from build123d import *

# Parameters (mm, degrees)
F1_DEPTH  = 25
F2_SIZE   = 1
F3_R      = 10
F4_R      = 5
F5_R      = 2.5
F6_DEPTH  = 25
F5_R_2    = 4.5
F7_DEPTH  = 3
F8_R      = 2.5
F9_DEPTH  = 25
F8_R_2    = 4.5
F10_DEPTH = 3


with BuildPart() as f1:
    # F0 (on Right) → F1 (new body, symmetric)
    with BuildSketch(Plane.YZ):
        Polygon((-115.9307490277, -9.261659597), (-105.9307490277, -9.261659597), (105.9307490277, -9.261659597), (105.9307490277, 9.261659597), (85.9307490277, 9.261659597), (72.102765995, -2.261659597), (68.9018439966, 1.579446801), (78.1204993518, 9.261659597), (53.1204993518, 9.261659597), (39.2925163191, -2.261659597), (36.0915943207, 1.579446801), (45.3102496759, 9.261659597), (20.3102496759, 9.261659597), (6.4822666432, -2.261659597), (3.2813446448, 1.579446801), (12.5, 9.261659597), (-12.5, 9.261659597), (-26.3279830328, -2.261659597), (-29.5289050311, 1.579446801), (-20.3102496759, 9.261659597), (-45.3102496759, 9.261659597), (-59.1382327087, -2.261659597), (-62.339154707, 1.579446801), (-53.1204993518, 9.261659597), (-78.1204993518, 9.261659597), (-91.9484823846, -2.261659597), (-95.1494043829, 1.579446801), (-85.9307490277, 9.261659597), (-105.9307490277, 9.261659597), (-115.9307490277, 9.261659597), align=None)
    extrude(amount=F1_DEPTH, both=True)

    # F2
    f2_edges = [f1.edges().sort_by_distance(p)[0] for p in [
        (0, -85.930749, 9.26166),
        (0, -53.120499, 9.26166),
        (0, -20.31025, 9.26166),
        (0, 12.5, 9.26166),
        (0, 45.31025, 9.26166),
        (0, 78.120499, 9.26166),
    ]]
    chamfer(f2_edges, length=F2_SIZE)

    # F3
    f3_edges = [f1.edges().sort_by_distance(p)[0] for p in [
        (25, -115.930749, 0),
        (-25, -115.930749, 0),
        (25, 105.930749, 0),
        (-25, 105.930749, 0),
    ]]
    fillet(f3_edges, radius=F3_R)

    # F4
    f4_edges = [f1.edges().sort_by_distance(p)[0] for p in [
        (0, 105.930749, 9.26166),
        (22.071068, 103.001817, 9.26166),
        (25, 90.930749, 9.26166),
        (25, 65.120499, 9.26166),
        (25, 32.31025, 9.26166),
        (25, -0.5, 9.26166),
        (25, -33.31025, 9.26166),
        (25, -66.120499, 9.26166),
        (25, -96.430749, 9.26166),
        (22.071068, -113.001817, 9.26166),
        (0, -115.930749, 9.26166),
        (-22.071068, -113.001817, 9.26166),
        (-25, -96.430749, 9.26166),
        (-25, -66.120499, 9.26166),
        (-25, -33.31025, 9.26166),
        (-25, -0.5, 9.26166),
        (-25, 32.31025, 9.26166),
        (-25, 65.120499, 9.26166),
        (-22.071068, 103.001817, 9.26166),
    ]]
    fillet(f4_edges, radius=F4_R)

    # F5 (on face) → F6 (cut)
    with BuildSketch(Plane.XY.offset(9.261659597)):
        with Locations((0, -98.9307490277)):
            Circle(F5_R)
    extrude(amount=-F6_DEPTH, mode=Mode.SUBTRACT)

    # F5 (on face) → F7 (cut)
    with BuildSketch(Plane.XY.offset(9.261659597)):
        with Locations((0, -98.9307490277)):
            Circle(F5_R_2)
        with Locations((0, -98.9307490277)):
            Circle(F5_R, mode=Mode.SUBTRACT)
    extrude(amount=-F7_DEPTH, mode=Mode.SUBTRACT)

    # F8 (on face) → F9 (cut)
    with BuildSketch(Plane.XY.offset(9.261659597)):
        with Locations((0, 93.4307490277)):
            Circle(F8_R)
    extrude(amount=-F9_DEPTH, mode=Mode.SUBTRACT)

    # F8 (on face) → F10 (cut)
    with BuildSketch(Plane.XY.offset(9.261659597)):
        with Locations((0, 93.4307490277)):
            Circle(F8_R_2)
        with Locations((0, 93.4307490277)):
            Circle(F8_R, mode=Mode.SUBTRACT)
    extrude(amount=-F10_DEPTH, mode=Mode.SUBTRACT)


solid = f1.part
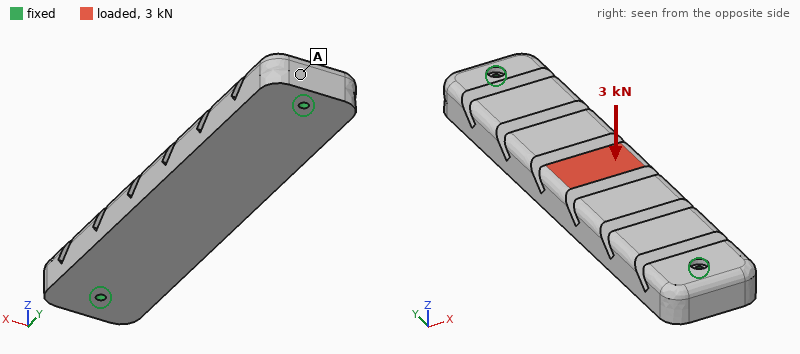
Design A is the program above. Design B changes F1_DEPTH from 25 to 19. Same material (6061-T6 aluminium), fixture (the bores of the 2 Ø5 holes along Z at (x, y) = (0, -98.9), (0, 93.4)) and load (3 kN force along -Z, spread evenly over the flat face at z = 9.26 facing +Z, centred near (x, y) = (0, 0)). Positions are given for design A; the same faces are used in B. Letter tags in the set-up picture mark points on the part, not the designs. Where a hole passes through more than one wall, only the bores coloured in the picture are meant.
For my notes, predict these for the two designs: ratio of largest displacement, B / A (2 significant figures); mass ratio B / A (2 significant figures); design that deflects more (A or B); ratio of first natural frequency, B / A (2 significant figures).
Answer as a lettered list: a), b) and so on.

a) 1.3
b) 0.75
c) B
d) 1.0
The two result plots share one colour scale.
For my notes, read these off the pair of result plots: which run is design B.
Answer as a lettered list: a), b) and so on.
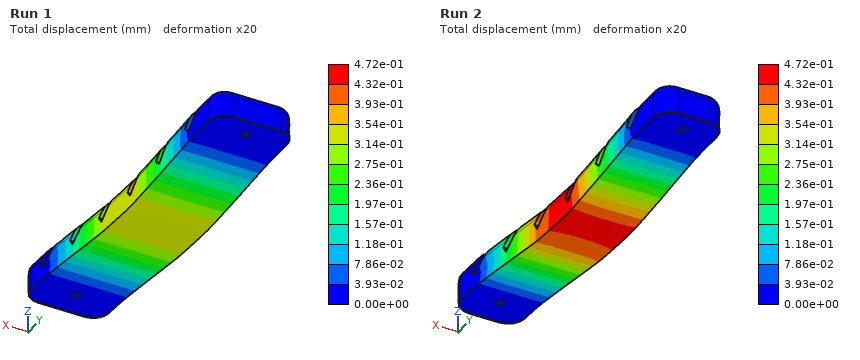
a) Run 2
